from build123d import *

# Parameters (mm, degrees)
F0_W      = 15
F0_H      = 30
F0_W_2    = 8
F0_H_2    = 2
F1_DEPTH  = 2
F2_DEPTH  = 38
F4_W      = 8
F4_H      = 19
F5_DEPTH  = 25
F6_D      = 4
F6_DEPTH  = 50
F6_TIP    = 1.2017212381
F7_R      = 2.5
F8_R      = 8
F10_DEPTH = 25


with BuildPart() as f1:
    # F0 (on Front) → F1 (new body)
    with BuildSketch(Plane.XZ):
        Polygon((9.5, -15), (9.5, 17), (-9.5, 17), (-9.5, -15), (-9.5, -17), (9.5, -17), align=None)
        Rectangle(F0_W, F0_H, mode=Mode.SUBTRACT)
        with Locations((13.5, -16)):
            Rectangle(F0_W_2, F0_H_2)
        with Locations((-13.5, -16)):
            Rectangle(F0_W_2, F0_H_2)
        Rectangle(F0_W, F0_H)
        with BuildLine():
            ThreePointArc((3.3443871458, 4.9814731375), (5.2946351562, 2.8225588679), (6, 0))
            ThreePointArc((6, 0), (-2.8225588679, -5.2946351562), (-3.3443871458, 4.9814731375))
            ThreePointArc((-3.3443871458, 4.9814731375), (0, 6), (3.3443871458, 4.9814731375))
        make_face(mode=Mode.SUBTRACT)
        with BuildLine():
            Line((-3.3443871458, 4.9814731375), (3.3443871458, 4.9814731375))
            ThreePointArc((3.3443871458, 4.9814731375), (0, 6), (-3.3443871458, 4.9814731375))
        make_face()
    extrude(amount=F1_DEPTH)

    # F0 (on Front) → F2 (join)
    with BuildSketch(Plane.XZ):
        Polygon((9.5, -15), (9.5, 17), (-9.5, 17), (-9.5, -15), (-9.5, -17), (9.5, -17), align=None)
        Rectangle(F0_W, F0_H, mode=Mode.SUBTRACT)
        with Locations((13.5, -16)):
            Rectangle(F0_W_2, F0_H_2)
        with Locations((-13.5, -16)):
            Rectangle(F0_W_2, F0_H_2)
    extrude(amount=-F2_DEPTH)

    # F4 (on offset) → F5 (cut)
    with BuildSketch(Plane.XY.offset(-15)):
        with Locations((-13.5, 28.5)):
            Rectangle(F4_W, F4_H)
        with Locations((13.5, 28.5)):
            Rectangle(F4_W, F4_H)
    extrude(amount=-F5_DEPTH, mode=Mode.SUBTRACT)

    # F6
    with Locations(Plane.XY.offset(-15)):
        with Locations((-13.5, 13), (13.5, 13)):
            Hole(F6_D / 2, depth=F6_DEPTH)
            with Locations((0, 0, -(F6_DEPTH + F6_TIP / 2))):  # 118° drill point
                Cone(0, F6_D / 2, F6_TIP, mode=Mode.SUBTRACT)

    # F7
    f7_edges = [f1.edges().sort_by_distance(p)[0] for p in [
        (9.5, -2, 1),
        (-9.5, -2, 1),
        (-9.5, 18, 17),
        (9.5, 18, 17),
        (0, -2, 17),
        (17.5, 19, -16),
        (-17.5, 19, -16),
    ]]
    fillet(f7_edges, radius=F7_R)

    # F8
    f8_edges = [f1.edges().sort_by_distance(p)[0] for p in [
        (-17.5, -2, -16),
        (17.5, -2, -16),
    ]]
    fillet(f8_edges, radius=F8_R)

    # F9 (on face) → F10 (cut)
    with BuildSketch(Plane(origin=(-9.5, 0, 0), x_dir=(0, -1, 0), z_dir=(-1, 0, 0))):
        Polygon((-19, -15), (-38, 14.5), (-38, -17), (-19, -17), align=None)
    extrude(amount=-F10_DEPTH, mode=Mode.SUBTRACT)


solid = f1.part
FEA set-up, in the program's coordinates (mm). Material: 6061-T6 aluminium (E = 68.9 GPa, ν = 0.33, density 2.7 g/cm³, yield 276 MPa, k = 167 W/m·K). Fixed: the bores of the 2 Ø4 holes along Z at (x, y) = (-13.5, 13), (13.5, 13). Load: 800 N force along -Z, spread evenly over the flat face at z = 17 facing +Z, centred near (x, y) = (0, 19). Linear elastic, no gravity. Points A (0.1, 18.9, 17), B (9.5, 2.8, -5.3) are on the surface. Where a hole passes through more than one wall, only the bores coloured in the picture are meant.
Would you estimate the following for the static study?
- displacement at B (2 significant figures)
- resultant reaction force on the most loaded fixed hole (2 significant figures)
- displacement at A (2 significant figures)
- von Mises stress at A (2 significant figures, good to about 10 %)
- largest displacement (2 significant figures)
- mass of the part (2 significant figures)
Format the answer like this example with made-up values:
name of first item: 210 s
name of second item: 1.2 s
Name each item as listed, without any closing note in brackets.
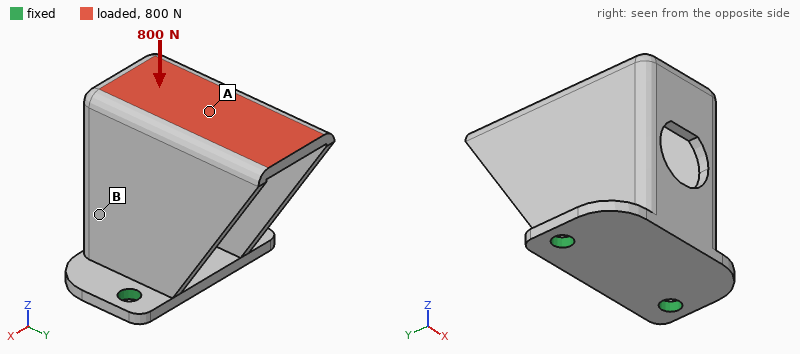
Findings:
displacement at B: 0.082 mm
resultant reaction force on the most loaded fixed hole: 400 N
displacement at A: 0.22 mm
von Mises stress at A: 41 MPa
largest displacement: 0.29 mm
mass of the part: 19 g
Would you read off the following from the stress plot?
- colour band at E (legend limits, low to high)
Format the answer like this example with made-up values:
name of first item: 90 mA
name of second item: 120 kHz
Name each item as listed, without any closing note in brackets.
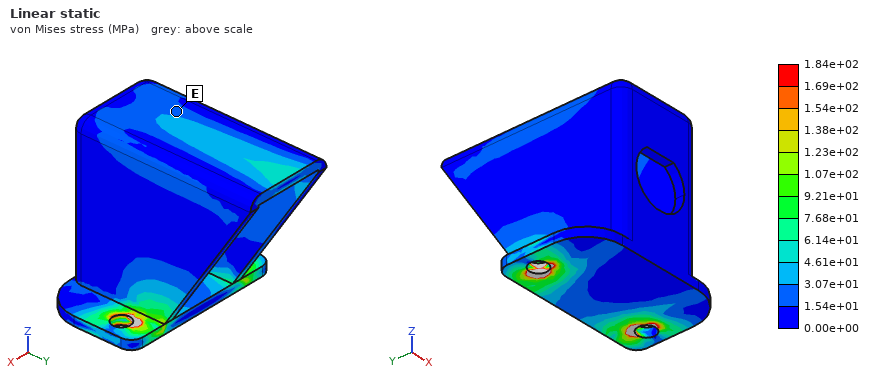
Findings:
colour band at E: 1.54e+01 to 3.07e+01 MPa
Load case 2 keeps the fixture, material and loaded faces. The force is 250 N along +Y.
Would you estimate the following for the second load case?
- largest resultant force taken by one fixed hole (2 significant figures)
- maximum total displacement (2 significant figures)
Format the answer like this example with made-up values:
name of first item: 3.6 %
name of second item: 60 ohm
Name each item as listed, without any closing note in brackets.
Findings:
largest resultant force taken by one fixed hole: 130 N
maximum total displacement: 0.41 mm
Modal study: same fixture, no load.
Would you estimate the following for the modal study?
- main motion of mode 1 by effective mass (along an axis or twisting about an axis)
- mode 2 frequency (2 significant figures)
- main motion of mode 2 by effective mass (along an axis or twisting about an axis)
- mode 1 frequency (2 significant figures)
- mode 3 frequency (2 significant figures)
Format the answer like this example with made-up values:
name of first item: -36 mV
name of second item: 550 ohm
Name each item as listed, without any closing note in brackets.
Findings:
main motion of mode 1 by effective mass: along Y
mode 2 frequency: 1600 Hz
main motion of mode 2 by effective mass: along X
mode 1 frequency: 1400 Hz
mode 3 frequency: 6700 Hz
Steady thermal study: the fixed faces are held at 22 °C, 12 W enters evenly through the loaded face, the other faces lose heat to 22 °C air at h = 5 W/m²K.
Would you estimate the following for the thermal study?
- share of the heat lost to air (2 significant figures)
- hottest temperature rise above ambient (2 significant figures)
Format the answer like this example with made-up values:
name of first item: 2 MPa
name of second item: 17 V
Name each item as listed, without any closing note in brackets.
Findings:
share of the heat lost to air: 4.3 %
hottest temperature rise above ambient: 28 K
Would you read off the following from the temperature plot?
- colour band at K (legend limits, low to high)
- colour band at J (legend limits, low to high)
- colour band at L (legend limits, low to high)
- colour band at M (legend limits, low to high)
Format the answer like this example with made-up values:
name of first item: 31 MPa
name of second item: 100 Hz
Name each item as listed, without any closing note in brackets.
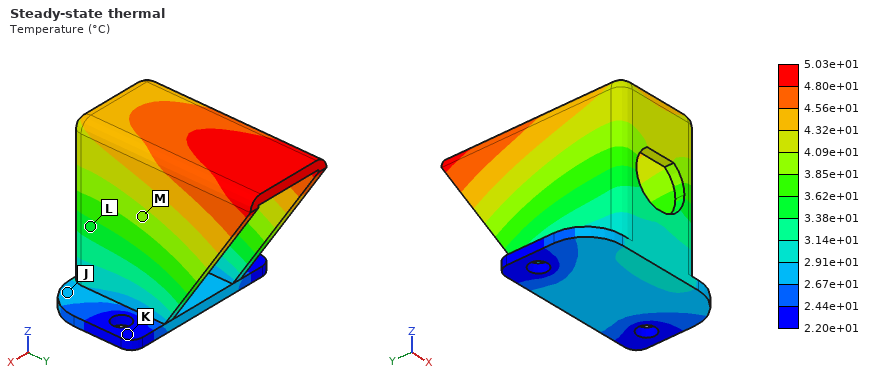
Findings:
colour band at K: 2.20e+01 to 2.44e+01 °C
colour band at J: 2.67e+01 to 2.91e+01 °C
colour band at L: 3.38e+01 to 3.62e+01 °C
colour band at M: 3.85e+01 to 4.09e+01 °C
